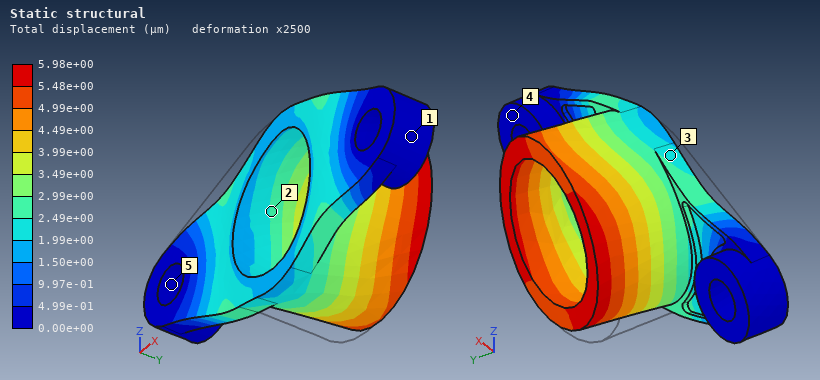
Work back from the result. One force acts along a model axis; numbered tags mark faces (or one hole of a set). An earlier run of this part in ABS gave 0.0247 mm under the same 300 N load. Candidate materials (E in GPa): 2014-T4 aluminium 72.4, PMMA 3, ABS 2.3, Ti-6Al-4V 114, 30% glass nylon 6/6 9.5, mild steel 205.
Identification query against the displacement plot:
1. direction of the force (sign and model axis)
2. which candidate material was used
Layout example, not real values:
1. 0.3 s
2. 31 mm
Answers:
1. +X
2. 30% glass nylon 6/6
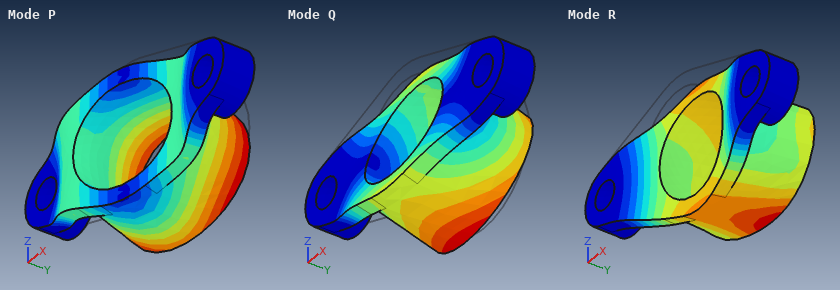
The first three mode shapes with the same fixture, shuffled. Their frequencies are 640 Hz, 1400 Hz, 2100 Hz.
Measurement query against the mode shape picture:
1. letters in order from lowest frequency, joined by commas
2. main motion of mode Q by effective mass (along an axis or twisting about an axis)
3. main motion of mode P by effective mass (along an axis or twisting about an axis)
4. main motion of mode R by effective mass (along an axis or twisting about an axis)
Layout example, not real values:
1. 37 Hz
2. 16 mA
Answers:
1. Q, R, P
2. along Z
3. along X
4. along Y
